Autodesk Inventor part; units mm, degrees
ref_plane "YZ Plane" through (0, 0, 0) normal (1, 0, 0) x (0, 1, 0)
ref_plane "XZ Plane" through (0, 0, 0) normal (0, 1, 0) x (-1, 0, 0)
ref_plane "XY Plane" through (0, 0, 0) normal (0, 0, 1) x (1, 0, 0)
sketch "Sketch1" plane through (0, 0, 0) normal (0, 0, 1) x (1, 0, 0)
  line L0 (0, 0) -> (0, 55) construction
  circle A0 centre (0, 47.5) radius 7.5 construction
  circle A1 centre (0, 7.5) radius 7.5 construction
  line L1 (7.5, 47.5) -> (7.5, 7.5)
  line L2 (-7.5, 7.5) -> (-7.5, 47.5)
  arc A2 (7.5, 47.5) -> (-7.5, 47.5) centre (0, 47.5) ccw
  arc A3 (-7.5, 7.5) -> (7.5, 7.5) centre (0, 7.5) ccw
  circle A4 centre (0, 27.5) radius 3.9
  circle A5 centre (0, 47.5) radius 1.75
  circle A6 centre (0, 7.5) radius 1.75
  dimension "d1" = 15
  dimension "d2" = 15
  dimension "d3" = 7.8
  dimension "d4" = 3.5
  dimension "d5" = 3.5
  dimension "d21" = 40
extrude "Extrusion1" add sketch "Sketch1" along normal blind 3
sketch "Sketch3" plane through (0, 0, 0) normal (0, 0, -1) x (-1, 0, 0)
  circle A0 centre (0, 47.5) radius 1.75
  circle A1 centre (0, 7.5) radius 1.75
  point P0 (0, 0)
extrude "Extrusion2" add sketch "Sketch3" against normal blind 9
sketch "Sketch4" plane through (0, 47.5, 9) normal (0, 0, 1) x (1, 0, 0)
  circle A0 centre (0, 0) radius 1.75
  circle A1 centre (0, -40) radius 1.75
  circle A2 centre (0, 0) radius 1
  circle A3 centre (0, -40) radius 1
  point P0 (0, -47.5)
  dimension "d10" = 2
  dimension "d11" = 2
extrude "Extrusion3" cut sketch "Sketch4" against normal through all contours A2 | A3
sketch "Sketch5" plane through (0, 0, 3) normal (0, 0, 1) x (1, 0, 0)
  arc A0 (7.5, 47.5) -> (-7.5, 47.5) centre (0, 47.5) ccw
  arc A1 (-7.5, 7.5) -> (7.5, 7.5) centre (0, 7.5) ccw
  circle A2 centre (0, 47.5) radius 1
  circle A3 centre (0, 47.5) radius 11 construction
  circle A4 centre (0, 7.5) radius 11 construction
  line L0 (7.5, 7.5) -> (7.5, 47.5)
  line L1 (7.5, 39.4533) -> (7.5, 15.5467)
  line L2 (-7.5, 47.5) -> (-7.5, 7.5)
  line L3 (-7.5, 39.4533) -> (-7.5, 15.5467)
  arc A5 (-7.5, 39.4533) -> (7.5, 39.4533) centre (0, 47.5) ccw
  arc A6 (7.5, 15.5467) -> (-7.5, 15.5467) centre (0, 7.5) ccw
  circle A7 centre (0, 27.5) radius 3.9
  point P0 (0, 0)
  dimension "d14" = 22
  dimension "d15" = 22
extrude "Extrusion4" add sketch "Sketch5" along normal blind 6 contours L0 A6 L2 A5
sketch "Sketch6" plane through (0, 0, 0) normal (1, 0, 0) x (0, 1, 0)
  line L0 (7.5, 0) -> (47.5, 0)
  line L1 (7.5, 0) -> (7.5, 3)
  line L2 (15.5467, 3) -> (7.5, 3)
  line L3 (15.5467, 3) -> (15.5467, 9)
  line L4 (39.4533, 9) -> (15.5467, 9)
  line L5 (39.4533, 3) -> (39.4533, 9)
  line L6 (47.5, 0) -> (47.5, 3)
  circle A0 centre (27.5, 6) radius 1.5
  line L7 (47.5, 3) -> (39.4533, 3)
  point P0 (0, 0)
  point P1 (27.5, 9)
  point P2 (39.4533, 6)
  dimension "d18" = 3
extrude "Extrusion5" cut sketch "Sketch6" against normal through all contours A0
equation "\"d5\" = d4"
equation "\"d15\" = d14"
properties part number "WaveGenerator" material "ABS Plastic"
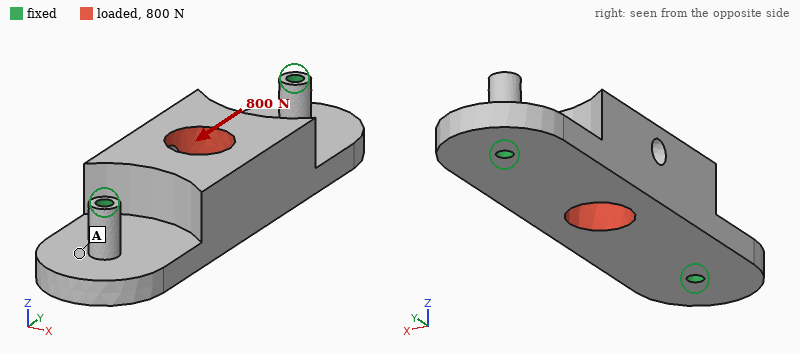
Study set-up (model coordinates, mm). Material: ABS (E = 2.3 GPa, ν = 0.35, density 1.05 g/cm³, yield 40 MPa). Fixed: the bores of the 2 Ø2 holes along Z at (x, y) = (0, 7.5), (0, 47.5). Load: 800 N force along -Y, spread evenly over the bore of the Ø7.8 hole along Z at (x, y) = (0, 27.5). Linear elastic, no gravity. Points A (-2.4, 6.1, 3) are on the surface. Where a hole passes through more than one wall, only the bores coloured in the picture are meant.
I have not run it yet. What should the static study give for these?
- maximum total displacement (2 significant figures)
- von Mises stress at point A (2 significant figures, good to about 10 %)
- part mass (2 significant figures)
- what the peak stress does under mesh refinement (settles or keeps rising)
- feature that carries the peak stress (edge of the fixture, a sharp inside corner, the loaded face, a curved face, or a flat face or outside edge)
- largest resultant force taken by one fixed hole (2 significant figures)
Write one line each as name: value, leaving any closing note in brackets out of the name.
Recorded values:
maximum total displacement: 0.20 mm
von Mises stress at point A: 5.2 MPa
part mass: 3.9 g
what the peak stress does under mesh refinement: keeps rising
feature that carries the peak stress: edge of the fixture
largest resultant force taken by one fixed hole: 410 N
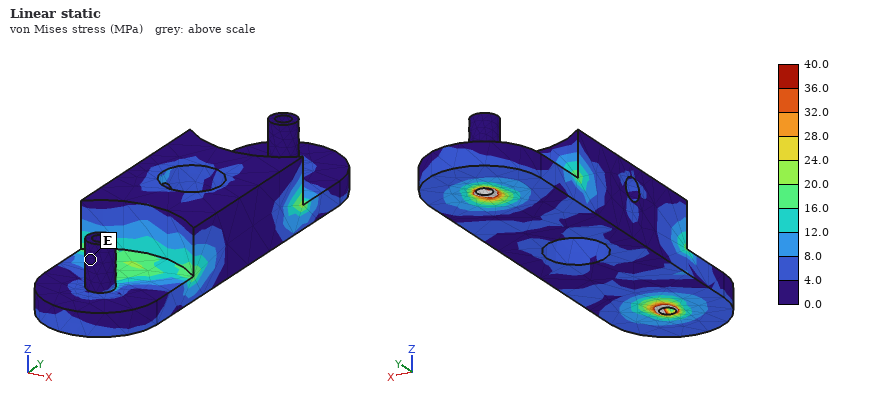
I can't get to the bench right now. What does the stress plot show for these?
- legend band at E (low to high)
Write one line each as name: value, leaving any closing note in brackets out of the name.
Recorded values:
legend band at E: 0.0 to 4.0 MPa
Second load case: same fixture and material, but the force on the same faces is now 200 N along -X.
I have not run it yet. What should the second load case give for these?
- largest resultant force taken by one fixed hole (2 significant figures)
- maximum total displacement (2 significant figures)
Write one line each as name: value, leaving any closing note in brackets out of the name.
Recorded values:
largest resultant force taken by one fixed hole: 100 N
maximum total displacement: 0.38 mm
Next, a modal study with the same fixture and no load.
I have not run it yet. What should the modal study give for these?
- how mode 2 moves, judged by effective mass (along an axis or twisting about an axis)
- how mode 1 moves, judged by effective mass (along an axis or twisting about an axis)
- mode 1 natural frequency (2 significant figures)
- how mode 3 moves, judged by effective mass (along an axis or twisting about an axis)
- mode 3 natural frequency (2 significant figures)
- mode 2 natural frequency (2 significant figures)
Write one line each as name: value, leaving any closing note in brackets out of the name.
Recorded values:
how mode 2 moves, judged by effective mass: along Z
how mode 1 moves, judged by effective mass: along X
mode 1 natural frequency: 2300 Hz
how mode 3 moves, judged by effective mass: along X
mode 3 natural frequency: 5300 Hz
mode 2 natural frequency: 2700 Hz
